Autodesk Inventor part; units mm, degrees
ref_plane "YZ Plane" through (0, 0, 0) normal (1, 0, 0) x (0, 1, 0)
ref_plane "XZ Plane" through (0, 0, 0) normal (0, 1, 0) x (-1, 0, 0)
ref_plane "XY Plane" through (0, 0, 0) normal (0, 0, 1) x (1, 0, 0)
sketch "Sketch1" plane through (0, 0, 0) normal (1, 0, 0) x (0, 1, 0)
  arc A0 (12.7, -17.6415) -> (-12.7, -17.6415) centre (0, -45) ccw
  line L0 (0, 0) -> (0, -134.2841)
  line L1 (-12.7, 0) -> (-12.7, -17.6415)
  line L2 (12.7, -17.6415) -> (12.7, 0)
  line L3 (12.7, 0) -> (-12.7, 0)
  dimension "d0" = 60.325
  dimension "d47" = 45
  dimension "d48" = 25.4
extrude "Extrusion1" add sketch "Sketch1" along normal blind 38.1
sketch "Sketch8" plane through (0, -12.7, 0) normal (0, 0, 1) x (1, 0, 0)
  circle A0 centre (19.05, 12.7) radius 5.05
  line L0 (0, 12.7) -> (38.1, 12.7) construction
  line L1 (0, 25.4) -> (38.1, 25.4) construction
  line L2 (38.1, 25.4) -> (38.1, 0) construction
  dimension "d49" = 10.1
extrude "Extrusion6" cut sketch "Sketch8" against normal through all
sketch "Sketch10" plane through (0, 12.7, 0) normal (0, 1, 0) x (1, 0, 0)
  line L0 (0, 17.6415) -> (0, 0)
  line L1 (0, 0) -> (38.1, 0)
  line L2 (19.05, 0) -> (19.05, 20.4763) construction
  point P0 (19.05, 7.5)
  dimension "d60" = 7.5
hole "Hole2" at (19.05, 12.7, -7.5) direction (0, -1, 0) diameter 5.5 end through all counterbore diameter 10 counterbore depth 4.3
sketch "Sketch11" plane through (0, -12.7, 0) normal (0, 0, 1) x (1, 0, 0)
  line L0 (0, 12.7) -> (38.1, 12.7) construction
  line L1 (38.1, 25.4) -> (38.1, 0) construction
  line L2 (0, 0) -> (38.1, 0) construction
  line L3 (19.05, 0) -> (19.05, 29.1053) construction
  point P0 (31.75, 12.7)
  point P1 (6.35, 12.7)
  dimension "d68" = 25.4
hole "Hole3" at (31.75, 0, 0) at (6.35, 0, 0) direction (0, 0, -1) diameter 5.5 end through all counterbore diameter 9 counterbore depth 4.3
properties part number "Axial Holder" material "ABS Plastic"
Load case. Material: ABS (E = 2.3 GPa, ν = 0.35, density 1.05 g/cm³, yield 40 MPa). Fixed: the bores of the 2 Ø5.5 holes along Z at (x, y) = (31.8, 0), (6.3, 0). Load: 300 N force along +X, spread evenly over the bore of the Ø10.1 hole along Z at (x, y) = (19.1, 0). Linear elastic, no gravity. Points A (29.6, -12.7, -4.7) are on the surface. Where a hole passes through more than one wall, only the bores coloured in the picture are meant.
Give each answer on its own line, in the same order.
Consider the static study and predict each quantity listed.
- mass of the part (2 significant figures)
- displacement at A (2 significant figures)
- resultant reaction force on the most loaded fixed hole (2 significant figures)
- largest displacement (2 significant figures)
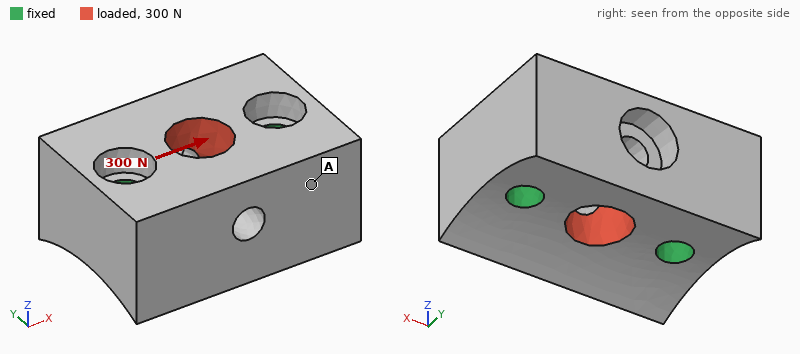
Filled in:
13 g
3.4 µm
150 N
7.5 µm
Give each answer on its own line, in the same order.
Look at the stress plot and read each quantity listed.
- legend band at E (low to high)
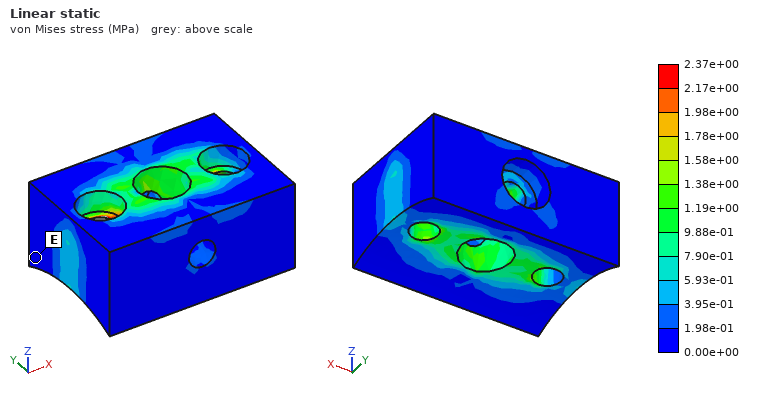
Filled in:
0.00e+00 to 1.98e-01 MPa
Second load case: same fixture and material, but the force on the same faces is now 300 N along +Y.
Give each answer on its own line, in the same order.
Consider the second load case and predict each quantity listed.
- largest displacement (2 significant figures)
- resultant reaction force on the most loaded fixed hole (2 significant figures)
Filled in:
13 µm
150 N
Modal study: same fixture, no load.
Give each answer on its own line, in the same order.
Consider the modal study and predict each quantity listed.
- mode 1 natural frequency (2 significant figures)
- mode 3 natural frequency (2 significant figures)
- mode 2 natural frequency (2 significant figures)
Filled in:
7900 Hz
11 kHz
10 kHz
